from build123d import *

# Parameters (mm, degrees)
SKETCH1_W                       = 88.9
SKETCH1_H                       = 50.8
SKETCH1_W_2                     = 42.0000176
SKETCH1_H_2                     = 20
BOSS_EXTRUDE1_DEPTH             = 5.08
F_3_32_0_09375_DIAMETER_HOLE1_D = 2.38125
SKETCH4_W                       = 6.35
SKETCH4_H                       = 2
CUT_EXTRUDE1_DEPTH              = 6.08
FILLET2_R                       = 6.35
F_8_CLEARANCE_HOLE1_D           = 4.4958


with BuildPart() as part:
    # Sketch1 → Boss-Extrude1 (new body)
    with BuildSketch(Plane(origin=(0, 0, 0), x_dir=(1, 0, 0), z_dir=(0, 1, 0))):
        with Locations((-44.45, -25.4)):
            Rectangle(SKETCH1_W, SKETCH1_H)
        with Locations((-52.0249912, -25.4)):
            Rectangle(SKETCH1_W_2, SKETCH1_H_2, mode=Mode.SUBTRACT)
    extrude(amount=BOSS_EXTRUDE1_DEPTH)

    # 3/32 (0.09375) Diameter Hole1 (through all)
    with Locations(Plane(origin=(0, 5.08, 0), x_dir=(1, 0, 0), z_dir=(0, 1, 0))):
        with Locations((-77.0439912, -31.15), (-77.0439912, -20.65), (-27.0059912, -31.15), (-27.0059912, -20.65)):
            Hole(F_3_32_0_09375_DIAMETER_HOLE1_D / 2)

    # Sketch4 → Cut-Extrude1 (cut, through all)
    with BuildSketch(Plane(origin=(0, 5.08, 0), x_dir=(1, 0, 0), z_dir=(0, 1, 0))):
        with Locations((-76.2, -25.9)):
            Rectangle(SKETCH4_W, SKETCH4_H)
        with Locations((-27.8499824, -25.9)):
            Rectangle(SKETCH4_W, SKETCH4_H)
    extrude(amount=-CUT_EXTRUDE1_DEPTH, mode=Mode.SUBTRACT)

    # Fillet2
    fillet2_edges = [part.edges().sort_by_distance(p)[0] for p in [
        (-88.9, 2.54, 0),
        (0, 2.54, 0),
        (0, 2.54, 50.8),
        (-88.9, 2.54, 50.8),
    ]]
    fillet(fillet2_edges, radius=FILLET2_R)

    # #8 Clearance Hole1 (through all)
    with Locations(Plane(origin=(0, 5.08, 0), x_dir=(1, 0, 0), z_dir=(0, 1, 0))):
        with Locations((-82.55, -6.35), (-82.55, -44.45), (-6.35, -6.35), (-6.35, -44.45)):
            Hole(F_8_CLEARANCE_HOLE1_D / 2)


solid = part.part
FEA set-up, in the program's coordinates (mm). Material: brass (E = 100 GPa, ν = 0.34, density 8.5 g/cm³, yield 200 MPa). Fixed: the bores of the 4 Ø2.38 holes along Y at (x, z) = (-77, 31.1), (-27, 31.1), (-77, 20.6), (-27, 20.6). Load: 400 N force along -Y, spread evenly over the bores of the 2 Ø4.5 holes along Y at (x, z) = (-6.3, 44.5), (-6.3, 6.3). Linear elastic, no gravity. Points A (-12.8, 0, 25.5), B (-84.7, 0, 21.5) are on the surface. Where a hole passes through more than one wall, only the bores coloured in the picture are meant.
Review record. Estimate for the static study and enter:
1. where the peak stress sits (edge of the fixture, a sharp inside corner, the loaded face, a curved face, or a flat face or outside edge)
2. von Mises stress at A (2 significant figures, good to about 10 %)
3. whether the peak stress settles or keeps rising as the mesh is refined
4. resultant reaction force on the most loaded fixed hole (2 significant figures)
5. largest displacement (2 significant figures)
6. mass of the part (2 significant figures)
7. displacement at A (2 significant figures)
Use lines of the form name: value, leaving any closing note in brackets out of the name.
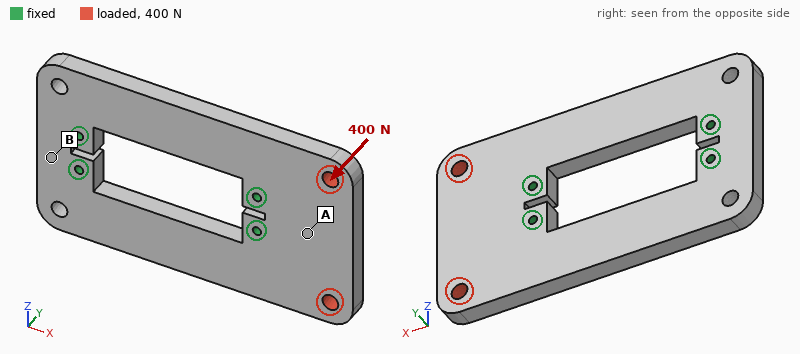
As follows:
where the peak stress sits: edge of the fixture
von Mises stress at A: 18 MPa
whether the peak stress settles or keeps rising as the mesh is refined: keeps rising
resultant reaction force on the most loaded fixed hole: 230 N
largest displacement: 54 µm
mass of the part: 150 g
displacement at A: 18 µm
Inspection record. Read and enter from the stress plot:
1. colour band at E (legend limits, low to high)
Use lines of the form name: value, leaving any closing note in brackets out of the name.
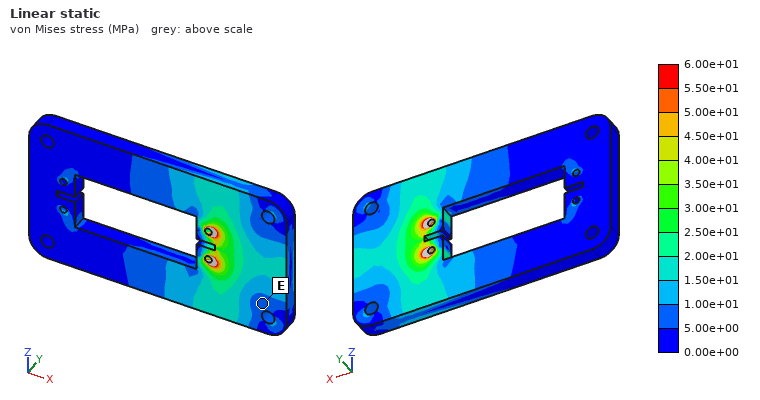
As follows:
colour band at E: 5.00e+00 to 1.00e+01 MPa
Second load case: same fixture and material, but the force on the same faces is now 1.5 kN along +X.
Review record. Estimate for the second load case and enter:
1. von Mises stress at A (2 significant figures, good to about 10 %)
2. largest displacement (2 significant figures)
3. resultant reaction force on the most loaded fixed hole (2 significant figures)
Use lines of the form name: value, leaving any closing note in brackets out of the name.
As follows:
von Mises stress at A: 3.7 MPa
largest displacement: 4.7 µm
resultant reaction force on the most loaded fixed hole: 630 N
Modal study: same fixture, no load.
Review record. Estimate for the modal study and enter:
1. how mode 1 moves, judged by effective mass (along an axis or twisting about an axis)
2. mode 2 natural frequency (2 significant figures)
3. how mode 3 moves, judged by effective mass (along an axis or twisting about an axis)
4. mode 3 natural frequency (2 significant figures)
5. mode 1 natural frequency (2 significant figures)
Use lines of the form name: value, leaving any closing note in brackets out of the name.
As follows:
how mode 1 moves, judged by effective mass: twisting about Z
mode 2 natural frequency: 3400 Hz
how mode 3 moves, judged by effective mass: along Y
mode 3 natural frequency: 3700 Hz
mode 1 natural frequency: 3000 Hz
